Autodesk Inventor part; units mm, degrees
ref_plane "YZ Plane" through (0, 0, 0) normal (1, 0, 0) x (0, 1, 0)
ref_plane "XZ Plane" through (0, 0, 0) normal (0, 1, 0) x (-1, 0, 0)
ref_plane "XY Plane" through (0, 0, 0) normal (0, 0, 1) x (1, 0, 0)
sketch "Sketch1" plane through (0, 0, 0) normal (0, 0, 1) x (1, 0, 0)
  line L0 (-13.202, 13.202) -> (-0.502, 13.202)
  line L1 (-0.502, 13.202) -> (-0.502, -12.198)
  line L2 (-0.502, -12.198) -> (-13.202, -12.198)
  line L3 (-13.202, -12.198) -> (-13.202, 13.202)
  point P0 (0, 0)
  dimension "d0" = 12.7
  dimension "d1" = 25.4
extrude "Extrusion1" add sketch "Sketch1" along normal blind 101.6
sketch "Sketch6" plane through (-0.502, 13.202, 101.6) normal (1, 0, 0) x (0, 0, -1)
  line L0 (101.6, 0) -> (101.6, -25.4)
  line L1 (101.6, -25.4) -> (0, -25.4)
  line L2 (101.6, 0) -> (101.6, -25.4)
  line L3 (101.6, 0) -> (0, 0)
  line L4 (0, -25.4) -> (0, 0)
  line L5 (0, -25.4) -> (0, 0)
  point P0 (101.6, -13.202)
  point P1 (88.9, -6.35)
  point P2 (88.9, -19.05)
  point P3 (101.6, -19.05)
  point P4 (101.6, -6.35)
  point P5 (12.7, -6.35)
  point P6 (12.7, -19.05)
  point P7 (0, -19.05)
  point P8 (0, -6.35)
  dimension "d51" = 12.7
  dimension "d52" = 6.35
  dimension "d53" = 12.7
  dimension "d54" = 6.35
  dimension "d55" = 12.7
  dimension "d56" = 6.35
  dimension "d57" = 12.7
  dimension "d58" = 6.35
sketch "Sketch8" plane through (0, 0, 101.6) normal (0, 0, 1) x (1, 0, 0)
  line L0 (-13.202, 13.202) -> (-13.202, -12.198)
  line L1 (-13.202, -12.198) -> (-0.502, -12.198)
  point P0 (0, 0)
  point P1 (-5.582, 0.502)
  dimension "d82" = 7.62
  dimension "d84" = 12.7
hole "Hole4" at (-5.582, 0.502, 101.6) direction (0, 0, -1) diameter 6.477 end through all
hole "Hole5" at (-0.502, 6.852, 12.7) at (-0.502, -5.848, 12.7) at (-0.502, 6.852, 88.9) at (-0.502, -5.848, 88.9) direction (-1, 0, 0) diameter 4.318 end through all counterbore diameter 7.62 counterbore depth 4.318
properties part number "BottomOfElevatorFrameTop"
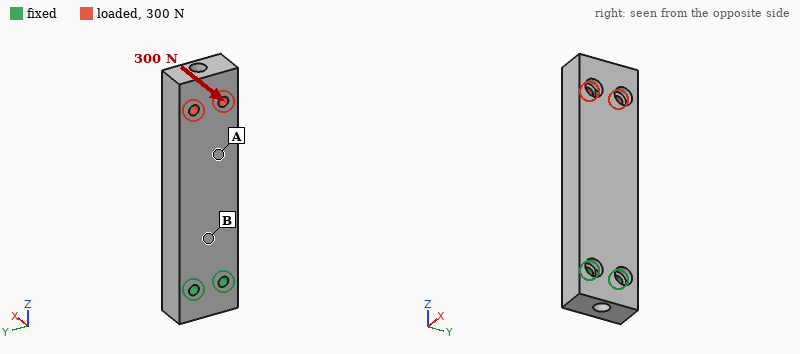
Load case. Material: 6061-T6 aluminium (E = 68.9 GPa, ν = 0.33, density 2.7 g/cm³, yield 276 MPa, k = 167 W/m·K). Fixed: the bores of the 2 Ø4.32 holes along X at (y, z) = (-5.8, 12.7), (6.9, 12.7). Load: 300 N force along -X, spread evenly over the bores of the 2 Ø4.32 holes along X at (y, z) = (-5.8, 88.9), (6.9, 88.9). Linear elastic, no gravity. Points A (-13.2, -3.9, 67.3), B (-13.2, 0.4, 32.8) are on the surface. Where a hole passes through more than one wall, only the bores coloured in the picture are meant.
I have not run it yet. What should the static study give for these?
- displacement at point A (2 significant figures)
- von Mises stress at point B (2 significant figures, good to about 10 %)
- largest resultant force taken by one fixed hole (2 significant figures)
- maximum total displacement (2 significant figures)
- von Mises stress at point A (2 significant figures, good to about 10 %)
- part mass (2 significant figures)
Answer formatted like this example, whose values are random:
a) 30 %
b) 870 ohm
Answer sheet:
a) 0.13 mm
b) 25 MPa
c) 180 N
d) 0.25 mm
e) 9.7 MPa
f) 76 g
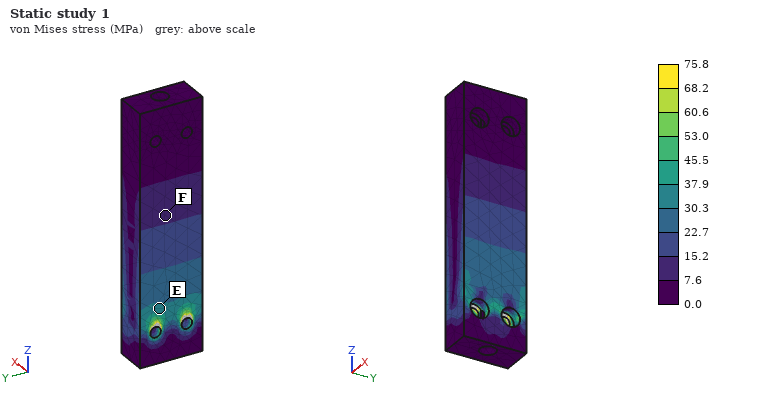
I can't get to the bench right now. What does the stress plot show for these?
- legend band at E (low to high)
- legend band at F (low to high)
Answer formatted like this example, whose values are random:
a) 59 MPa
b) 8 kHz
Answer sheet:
a) 30.3 to 37.9 MPa
b) 7.6 to 15.2 MPa
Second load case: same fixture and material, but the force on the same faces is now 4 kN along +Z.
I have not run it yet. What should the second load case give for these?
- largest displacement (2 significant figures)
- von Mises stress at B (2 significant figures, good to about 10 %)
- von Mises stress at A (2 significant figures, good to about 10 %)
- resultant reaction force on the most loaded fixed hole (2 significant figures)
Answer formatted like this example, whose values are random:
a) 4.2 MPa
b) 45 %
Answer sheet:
a) 99 µm
b) 26 MPa
c) 26 MPa
d) 2.0 kN
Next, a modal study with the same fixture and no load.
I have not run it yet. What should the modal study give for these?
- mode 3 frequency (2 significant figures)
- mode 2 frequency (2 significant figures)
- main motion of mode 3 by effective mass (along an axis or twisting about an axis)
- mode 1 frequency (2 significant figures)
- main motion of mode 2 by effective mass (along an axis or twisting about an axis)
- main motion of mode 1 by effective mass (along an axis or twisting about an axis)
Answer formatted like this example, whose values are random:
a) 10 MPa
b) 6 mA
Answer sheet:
a) 6300 Hz
b) 2400 Hz
c) twisting about Z
d) 1200 Hz
e) along Y
f) along X
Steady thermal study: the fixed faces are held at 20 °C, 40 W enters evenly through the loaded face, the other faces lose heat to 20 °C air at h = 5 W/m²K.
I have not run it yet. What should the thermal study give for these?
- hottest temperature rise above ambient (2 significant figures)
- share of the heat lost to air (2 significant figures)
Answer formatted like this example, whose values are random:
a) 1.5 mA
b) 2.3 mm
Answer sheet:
a) 66 K
b) 4.2 %
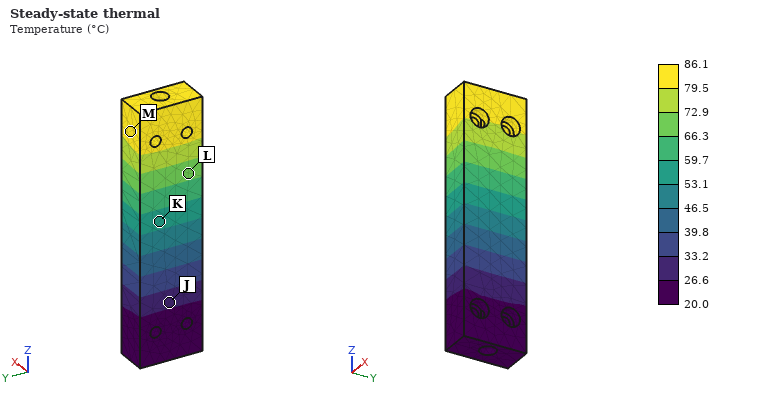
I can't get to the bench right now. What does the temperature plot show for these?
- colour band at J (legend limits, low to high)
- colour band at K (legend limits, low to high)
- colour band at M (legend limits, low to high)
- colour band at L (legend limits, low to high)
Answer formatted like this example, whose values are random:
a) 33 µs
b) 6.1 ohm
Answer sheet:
a) 26.6 to 33.2 °C
b) 53.1 to 59.7 °C
c) 79.5 to 86.1 °C
d) 66.3 to 72.9 °C
